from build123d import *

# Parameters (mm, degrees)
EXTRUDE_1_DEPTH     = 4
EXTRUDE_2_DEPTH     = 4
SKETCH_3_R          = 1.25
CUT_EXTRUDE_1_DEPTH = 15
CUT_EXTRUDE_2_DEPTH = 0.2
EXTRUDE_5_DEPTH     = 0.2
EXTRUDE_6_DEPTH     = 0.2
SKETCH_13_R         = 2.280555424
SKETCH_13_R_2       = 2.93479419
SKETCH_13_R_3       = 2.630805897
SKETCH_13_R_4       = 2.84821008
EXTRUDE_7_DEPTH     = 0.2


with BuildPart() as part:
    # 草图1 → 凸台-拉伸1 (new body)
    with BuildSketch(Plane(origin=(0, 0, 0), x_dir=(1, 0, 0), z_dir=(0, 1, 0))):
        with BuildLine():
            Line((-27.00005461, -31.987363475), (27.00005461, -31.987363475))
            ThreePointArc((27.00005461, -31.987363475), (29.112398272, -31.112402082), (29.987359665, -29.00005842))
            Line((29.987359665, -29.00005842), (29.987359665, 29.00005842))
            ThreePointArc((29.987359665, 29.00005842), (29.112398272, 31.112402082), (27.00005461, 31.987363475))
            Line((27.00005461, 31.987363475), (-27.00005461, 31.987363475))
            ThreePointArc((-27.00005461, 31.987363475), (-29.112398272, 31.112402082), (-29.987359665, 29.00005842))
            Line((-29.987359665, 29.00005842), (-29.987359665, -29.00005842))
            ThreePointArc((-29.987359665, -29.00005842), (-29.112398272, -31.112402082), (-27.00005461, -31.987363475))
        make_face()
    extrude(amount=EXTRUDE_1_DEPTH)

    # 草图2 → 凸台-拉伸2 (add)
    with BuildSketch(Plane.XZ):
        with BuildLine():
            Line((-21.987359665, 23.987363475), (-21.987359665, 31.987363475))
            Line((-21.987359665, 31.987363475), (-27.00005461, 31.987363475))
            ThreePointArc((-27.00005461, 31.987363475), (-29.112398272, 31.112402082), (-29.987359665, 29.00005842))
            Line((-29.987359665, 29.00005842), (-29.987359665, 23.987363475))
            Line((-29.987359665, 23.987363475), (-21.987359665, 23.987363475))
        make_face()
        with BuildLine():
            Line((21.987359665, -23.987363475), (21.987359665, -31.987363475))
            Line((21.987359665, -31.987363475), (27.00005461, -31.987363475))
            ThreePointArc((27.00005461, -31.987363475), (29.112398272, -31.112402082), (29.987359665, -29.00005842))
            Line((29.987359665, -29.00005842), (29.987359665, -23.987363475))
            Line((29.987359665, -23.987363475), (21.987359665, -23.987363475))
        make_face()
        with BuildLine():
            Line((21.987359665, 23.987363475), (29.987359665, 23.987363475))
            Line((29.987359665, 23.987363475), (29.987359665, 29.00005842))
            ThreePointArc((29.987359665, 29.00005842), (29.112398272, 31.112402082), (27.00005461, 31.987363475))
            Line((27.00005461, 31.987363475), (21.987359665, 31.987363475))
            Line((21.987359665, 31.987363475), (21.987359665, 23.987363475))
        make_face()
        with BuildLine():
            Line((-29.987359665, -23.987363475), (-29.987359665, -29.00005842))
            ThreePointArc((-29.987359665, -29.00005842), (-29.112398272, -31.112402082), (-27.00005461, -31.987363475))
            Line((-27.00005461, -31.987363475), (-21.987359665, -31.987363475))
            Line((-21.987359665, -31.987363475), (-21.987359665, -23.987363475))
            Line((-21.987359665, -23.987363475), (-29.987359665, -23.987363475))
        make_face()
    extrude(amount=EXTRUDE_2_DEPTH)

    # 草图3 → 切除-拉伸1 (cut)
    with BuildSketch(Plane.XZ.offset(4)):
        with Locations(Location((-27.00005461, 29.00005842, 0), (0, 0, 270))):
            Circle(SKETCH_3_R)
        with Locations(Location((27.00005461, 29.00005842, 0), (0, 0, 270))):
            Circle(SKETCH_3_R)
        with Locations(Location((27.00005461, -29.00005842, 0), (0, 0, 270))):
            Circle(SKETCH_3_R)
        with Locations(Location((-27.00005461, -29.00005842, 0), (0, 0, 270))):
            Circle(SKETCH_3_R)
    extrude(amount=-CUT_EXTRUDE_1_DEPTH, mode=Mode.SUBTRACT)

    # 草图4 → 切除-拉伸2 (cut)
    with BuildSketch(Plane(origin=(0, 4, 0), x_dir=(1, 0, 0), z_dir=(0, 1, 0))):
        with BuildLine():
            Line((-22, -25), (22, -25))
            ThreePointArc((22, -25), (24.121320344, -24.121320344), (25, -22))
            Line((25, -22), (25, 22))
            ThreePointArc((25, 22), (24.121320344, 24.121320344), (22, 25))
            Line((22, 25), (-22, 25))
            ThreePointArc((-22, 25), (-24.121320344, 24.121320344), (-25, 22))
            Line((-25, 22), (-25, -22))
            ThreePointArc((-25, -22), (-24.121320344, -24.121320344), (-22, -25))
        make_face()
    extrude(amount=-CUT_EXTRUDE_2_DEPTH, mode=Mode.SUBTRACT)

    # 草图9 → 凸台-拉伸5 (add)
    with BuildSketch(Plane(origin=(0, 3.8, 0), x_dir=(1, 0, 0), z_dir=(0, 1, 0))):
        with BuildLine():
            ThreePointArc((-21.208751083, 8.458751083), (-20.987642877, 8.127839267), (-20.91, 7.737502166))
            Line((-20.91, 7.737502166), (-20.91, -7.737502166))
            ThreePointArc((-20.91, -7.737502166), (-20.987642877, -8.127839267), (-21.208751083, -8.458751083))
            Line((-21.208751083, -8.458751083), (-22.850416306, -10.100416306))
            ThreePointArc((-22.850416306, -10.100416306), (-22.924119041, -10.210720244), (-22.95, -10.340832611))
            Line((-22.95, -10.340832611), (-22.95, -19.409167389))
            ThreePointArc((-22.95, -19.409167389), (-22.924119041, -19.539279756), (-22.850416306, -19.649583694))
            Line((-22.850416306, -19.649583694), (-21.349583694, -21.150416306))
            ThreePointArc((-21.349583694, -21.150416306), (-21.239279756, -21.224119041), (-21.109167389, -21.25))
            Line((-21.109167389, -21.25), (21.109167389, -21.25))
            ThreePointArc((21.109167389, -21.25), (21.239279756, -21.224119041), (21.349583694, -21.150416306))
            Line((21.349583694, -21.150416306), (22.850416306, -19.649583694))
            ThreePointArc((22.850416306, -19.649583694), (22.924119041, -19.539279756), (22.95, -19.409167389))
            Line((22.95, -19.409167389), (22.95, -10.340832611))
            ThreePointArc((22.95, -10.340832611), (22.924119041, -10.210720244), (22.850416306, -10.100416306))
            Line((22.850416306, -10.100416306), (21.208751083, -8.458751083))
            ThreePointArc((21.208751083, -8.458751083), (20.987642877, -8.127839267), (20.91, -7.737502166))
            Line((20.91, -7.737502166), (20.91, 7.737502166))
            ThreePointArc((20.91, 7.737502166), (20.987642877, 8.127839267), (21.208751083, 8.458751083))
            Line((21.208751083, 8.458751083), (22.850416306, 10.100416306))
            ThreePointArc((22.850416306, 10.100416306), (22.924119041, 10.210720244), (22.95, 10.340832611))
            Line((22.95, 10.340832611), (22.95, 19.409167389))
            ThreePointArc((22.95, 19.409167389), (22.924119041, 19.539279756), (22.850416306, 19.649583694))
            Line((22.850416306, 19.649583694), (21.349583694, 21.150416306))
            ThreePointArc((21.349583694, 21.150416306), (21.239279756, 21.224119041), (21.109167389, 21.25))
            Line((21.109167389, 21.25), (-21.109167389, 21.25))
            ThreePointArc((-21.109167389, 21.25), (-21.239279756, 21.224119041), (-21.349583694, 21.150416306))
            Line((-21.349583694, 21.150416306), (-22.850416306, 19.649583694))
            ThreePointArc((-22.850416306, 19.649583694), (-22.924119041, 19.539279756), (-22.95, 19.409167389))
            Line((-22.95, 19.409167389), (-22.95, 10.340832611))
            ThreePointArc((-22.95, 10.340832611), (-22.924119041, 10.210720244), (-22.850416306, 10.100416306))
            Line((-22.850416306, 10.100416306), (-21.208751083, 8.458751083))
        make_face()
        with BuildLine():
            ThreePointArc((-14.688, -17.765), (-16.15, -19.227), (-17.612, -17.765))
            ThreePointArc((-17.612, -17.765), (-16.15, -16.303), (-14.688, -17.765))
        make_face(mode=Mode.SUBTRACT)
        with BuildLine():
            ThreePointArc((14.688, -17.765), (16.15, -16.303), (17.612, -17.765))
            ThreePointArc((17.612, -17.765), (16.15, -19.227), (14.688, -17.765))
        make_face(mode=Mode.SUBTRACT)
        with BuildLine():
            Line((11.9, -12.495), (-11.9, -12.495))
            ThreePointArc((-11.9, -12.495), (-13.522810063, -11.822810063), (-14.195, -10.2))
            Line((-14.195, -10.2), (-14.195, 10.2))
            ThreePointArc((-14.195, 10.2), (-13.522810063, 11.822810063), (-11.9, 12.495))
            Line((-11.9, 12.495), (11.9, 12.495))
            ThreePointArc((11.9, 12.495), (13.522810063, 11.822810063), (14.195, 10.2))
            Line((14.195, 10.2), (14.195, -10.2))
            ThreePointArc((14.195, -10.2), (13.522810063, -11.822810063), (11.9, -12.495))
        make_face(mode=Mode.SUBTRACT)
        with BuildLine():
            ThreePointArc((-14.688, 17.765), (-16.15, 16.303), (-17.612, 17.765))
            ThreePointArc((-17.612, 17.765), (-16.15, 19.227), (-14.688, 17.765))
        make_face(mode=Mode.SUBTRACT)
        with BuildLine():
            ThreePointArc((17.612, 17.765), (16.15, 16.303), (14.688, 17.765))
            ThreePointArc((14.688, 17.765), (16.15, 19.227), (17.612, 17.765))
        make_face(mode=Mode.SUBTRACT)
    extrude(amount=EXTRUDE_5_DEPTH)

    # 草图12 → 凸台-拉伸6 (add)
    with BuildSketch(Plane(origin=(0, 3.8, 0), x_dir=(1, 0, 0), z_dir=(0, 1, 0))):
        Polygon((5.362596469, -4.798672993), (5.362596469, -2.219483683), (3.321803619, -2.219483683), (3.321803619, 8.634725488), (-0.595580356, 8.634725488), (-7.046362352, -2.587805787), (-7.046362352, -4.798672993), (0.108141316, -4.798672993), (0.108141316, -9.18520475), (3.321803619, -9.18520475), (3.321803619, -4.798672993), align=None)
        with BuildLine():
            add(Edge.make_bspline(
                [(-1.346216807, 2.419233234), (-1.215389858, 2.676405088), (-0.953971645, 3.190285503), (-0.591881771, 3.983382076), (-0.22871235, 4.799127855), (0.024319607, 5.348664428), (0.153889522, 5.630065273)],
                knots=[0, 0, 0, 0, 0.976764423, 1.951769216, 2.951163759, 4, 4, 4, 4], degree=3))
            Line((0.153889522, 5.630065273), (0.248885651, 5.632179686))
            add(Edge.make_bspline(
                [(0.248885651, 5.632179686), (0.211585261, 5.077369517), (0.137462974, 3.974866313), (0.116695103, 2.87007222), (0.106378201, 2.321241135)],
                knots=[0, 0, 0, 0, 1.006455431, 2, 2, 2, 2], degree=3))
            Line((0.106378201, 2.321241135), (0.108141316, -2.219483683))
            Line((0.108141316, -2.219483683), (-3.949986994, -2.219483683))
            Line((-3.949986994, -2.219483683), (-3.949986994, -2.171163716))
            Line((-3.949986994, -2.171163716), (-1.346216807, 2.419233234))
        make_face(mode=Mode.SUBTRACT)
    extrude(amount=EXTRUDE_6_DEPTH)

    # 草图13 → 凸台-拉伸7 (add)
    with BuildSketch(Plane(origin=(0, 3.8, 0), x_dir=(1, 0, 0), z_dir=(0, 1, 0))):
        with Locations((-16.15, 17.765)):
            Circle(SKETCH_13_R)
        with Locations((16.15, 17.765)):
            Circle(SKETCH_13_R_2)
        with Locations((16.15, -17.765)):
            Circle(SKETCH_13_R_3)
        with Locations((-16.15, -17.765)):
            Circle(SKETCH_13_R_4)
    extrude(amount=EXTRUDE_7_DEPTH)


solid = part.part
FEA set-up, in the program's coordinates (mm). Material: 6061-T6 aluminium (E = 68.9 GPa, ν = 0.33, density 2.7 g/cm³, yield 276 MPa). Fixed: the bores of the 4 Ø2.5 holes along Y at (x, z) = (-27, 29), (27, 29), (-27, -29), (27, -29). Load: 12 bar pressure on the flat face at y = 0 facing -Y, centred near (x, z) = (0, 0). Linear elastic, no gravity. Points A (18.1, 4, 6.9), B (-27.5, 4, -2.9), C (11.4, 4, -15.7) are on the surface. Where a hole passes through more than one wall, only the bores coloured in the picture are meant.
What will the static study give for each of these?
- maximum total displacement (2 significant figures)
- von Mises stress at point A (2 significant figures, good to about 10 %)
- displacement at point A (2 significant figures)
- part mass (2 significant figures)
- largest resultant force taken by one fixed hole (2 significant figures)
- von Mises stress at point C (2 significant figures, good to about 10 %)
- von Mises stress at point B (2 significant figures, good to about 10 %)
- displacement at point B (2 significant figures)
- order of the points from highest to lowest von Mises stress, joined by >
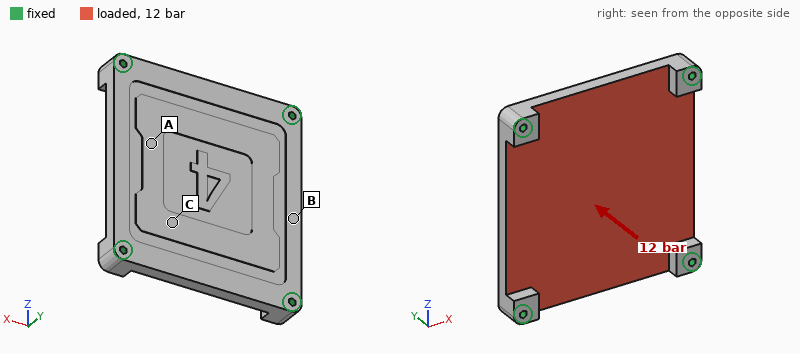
0.19 mm
66 MPa
0.14 mm
43 g
1.2 kN
43 MPa
83 MPa
0.11 mm
B > A > C
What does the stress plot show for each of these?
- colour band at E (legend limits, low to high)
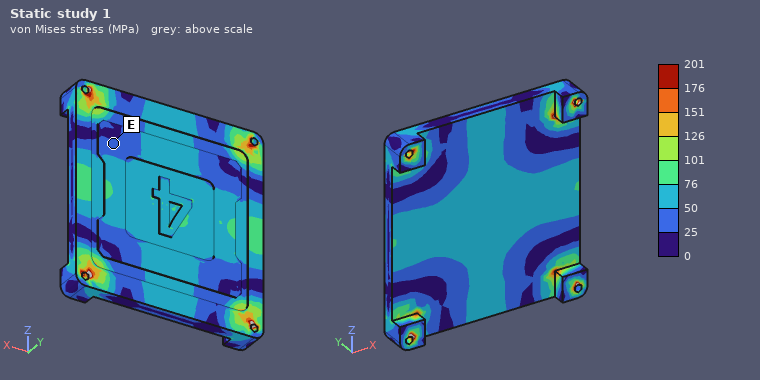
25 to 50 MPa
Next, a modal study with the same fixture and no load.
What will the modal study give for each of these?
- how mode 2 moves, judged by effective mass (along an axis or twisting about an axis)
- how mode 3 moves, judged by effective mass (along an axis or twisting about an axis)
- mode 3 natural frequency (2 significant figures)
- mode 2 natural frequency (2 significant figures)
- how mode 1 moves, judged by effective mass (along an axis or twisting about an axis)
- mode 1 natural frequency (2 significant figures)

twisting about Z
twisting about X
8400 Hz
7700 Hz
along Y
4700 Hz
